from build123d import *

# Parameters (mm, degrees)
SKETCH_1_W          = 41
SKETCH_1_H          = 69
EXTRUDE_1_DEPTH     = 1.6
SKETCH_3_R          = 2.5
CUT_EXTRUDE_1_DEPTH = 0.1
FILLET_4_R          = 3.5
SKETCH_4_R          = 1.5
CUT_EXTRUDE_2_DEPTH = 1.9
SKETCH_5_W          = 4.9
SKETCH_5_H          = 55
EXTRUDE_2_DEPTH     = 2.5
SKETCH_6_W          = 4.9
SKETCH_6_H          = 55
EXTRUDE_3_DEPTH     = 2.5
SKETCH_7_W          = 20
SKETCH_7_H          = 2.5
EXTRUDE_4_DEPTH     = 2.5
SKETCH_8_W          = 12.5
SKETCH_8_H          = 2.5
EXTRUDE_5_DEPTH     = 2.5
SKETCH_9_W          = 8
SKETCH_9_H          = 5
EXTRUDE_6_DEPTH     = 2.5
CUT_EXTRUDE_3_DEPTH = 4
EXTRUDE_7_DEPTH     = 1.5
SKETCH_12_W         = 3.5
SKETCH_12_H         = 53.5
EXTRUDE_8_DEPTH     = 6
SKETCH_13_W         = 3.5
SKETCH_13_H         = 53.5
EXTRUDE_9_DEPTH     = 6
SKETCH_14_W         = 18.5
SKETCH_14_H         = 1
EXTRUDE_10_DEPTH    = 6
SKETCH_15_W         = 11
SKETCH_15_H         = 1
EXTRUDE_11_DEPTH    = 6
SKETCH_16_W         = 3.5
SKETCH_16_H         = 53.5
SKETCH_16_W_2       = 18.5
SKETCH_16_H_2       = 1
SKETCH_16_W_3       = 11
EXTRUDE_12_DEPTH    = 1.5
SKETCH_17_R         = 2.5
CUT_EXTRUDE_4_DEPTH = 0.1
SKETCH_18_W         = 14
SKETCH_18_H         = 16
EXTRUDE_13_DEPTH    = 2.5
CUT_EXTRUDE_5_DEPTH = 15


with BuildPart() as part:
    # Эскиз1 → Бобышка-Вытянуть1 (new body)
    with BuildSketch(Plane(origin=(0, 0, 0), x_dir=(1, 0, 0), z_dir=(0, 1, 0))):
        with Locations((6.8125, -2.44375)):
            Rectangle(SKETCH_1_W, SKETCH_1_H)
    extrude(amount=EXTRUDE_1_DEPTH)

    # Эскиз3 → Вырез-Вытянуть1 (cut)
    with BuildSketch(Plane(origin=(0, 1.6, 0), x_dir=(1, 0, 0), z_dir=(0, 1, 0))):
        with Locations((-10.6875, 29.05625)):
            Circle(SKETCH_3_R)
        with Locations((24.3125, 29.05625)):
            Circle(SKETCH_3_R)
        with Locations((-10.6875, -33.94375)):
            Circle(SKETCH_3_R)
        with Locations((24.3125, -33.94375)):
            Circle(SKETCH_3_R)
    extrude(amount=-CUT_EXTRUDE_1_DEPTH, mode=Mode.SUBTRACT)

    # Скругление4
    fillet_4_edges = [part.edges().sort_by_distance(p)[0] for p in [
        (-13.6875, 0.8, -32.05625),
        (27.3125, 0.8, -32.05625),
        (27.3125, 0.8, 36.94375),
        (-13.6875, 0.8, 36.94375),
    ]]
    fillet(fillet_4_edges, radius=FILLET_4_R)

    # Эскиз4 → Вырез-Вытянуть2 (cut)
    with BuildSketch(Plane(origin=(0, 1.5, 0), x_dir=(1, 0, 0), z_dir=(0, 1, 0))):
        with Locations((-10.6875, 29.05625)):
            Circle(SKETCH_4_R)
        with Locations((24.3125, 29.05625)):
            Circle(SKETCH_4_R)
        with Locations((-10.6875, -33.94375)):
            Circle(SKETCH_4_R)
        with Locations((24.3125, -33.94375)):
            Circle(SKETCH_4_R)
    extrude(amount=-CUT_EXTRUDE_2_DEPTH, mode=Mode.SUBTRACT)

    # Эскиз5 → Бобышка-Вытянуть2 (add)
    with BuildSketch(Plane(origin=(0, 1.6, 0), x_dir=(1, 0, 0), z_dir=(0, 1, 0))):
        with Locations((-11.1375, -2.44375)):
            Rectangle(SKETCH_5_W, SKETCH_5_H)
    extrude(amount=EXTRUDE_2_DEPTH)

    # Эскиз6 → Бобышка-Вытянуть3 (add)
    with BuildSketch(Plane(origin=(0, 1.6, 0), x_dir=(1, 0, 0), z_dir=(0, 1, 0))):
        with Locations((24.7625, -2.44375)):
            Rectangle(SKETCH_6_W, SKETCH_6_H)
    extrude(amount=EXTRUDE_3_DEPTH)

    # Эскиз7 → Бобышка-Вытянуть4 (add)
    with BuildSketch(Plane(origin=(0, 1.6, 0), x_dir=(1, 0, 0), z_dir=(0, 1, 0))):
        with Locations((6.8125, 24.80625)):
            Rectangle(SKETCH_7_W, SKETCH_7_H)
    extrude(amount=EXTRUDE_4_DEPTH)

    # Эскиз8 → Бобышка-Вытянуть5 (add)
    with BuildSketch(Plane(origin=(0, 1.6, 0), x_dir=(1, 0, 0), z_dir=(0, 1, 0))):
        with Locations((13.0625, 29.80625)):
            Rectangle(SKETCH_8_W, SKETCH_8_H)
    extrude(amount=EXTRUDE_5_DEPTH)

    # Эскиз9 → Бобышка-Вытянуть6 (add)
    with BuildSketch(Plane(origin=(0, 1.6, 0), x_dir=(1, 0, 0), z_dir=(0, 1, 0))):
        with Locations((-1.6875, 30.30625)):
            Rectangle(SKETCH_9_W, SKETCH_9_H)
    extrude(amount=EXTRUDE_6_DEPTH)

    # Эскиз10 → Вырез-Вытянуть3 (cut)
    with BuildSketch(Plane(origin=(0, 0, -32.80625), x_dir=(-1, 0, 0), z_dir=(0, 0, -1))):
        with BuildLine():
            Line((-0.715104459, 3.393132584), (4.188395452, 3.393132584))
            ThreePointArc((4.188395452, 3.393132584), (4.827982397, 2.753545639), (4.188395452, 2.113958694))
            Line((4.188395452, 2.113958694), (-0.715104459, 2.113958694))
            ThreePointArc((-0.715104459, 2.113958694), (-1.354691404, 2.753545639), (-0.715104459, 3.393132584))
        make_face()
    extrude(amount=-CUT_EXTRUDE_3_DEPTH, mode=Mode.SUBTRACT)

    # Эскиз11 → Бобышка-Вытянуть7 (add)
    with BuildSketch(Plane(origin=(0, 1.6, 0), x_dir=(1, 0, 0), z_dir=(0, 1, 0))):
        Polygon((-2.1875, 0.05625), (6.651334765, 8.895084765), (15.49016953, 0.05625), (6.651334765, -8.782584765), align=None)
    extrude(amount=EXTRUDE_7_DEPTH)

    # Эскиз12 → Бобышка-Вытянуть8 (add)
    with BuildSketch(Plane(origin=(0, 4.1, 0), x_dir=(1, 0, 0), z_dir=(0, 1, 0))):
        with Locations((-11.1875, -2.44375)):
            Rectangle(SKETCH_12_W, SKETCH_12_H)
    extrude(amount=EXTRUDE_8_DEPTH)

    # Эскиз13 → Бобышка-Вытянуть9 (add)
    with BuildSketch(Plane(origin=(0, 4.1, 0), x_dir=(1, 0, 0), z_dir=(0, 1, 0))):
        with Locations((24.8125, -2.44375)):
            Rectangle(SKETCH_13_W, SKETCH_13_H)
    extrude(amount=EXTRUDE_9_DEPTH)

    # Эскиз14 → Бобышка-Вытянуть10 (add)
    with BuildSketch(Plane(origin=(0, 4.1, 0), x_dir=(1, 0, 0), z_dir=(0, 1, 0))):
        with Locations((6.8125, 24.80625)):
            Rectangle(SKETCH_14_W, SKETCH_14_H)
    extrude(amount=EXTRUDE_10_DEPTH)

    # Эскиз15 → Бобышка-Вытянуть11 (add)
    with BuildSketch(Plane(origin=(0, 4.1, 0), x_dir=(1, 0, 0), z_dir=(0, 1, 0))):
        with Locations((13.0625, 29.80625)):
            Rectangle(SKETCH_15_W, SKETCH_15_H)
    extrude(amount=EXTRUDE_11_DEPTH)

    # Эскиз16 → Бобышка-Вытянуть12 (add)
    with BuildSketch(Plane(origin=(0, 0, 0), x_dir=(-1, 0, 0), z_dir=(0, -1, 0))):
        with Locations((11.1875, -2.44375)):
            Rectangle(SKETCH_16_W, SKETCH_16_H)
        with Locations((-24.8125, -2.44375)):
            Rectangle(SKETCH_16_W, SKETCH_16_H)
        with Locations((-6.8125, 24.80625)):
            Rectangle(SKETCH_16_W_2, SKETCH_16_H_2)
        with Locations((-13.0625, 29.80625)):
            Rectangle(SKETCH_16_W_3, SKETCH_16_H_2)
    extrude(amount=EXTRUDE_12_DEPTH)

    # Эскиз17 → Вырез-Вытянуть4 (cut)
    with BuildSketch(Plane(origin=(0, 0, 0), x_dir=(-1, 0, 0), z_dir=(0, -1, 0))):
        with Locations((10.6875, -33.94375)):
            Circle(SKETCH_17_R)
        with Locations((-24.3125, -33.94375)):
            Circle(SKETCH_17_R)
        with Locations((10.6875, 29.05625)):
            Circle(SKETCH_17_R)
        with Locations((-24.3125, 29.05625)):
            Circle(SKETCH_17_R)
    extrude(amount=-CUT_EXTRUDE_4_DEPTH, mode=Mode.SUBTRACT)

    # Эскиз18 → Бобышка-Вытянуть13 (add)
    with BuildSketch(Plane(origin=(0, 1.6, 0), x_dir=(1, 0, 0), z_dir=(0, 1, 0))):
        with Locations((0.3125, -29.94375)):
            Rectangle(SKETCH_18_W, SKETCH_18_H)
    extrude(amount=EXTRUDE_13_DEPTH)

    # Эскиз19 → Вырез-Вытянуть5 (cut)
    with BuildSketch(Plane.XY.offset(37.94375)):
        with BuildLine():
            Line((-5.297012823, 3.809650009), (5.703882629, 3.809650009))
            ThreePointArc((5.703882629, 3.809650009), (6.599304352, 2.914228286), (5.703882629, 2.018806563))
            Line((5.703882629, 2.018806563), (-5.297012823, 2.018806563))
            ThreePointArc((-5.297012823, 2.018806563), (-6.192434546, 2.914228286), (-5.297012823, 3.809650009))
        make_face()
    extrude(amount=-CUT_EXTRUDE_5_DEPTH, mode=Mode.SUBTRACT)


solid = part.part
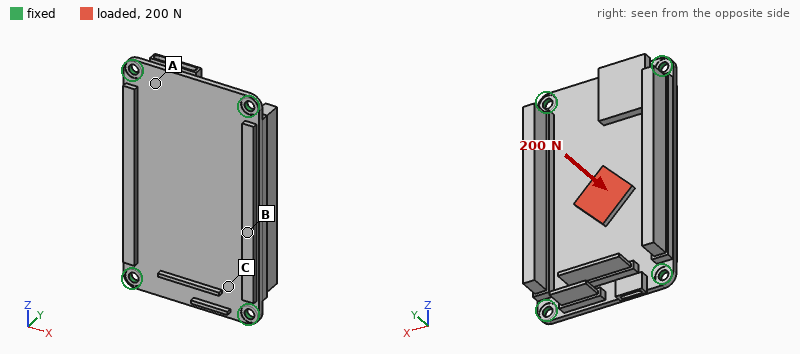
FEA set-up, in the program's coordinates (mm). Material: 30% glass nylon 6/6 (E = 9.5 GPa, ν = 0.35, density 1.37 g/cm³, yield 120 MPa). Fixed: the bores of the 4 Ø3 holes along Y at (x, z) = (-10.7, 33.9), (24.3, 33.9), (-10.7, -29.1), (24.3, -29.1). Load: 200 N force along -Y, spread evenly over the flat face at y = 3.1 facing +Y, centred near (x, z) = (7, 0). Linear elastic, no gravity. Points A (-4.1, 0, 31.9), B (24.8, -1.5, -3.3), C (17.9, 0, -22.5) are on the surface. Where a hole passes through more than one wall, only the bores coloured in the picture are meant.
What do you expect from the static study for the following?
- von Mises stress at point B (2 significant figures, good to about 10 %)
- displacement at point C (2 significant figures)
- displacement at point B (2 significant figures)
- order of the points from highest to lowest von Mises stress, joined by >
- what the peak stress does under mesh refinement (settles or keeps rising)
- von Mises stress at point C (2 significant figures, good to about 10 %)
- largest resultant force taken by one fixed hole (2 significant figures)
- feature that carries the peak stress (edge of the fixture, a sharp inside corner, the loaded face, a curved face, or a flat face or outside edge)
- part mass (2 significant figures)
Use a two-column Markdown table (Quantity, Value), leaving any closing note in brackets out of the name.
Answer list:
| Quantity | Value |
|---|---|
| von Mises stress at point B | 7.8 MPa |
| displacement at point C | 0.10 mm |
| displacement at point B | 0.081 mm |
| order of the points from highest to lowest von Mises stress, joined by > | C > B > A |
| what the peak stress does under mesh refinement | keeps rising |
| von Mises stress at point C | 15 MPa |
| largest resultant force taken by one fixed hole | 87 N |
| feature that carries the peak stress | edge of the fixture |
| part mass | 13 g |
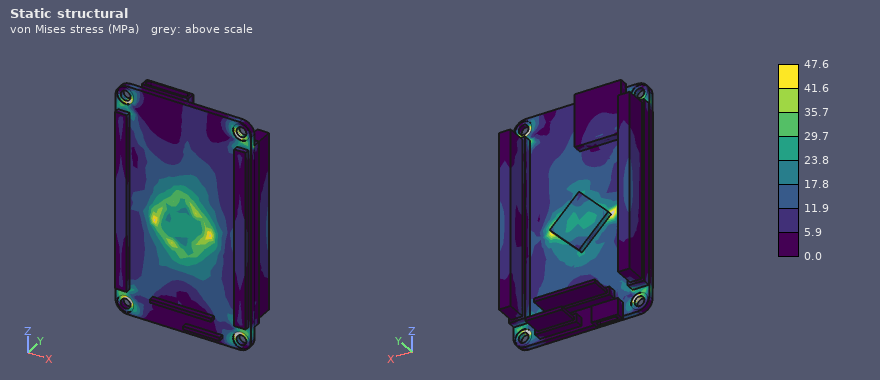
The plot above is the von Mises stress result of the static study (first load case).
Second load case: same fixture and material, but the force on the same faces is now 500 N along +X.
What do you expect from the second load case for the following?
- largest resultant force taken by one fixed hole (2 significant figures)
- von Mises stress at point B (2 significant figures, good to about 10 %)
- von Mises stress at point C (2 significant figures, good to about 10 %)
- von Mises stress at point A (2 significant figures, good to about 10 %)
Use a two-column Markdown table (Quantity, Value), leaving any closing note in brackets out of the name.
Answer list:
| Quantity | Value |
|---|---|
| largest resultant force taken by one fixed hole | 180 N |
| von Mises stress at point B | 7.8 MPa |
| von Mises stress at point C | 9.3 MPa |
| von Mises stress at point A | 6.4 MPa |
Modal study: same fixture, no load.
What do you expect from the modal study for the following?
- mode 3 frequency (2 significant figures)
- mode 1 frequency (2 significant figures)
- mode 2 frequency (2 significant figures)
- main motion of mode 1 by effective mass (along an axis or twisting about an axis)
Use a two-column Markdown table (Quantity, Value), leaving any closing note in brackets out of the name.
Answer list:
| Quantity | Value |
|---|---|
| mode 3 frequency | 3500 Hz |
| mode 1 frequency | 2200 Hz |
| mode 2 frequency | 3400 Hz |
| main motion of mode 1 by effective mass | along Y |
